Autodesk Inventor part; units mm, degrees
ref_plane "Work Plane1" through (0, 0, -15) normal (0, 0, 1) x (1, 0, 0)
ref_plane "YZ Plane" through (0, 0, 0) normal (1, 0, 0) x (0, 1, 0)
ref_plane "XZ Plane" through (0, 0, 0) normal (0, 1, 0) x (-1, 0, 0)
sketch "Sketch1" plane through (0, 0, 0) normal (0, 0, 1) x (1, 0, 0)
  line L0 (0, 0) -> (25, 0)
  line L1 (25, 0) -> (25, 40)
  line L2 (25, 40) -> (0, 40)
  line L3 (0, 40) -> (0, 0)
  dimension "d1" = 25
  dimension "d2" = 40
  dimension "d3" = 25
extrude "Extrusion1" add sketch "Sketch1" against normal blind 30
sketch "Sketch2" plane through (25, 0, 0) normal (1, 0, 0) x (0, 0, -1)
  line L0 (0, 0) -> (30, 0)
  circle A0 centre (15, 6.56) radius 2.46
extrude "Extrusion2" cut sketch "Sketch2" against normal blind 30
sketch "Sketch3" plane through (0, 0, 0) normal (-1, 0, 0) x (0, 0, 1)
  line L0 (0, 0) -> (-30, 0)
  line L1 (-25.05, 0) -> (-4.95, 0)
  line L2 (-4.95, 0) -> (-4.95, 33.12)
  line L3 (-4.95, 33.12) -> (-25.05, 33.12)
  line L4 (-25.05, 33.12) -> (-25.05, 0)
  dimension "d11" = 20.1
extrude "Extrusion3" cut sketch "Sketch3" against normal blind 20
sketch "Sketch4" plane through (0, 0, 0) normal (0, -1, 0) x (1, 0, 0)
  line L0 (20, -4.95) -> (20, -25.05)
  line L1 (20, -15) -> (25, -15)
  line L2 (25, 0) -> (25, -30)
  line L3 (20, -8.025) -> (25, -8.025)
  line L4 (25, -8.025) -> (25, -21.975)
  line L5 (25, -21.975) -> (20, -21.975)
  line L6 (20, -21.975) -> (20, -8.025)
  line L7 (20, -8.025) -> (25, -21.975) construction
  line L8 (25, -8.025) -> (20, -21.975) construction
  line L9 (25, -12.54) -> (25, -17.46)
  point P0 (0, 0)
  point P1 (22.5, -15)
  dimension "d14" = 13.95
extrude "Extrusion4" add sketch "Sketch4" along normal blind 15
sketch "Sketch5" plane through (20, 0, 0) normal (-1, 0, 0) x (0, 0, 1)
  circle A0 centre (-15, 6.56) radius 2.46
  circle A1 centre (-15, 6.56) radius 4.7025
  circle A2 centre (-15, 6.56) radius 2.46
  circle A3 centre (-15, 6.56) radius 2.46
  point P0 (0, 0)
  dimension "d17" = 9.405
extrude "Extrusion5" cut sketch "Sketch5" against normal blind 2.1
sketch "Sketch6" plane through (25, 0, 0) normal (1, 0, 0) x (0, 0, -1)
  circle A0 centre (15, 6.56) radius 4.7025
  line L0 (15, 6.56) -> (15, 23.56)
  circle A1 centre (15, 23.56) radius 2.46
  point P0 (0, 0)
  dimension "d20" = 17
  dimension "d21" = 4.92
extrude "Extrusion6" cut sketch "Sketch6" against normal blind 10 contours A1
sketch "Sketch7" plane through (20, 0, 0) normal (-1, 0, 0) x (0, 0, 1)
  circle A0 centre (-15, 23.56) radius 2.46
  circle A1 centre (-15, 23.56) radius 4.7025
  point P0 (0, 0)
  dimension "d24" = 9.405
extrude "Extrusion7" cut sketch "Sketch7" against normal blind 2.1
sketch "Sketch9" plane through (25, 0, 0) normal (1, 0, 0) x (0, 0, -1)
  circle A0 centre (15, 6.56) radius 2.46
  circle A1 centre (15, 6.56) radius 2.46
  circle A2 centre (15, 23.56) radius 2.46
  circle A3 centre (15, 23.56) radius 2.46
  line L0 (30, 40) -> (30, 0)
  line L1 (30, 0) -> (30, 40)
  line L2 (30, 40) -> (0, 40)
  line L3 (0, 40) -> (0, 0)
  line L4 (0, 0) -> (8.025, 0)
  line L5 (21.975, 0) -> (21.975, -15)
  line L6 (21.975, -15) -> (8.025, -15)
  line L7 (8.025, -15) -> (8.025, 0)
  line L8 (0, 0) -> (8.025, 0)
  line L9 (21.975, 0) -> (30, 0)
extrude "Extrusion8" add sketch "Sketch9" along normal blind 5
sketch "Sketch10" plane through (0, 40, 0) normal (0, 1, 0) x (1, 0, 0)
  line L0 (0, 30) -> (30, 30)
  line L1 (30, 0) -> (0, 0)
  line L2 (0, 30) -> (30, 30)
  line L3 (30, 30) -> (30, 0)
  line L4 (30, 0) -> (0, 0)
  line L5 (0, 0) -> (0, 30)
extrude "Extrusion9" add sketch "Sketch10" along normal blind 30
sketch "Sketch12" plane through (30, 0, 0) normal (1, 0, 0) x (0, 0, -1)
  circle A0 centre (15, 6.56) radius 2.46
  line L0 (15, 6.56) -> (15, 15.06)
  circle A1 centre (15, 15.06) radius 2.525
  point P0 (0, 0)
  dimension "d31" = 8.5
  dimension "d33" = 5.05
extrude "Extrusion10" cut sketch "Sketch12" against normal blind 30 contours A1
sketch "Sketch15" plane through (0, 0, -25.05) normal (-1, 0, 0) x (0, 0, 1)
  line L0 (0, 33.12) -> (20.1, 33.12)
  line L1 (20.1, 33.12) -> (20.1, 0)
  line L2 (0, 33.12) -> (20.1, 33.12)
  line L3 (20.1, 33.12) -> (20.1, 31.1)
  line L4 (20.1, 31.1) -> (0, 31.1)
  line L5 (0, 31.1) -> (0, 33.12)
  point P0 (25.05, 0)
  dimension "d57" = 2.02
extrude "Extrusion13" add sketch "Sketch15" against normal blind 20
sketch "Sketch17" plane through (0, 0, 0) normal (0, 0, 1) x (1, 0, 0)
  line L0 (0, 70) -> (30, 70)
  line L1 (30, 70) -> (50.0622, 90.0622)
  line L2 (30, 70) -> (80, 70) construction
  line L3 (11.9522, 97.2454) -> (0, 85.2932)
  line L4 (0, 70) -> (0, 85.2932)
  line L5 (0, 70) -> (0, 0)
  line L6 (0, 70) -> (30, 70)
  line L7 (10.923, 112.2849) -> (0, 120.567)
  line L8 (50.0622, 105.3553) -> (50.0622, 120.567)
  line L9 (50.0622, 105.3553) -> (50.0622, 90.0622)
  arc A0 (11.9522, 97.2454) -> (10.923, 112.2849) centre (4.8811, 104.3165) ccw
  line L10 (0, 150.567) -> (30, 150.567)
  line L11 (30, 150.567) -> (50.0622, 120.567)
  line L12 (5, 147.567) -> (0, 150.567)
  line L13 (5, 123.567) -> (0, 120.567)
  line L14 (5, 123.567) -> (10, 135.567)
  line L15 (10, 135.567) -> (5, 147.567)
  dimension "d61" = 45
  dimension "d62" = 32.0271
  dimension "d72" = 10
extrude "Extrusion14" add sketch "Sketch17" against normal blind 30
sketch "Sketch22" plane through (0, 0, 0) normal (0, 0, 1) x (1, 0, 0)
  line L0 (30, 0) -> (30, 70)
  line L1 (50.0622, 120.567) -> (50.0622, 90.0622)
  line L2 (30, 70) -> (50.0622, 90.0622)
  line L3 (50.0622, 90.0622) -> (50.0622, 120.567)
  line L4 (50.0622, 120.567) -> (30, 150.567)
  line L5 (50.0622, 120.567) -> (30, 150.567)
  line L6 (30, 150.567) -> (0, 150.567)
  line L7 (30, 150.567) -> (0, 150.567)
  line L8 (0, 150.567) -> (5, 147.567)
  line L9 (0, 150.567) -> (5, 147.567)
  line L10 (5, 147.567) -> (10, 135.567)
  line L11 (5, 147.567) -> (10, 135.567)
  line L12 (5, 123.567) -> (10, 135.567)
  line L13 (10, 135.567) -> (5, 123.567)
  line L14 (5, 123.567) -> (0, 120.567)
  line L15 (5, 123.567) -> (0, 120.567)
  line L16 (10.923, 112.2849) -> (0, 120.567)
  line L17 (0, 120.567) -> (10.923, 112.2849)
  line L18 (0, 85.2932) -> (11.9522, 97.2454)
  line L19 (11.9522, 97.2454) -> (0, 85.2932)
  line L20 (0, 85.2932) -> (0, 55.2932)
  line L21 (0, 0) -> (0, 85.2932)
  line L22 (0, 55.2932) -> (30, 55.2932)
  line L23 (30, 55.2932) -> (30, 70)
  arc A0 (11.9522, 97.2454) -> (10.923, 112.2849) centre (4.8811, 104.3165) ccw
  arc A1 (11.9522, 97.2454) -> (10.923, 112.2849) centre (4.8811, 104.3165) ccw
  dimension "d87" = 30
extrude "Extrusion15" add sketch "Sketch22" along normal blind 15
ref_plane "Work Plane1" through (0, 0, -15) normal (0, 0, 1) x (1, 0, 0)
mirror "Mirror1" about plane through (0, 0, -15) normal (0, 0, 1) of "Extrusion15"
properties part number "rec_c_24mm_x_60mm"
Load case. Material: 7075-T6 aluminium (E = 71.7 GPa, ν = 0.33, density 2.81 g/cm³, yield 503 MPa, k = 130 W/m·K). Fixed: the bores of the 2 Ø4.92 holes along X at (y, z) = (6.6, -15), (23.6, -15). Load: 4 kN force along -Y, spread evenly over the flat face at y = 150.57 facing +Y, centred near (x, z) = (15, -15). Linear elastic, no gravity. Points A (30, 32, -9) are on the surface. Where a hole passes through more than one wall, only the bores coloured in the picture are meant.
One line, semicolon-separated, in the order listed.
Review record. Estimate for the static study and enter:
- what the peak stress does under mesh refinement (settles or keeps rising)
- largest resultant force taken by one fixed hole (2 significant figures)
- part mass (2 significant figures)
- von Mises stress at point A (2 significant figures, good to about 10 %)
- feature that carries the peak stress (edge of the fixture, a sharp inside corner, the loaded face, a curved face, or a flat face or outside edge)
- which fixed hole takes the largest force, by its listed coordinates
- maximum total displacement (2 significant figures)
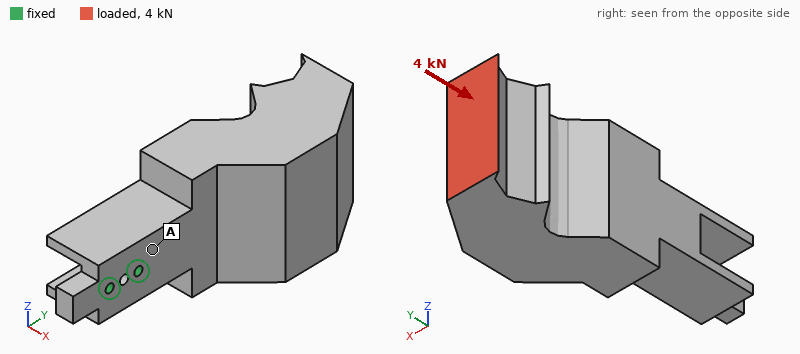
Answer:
keeps rising; 3.0 kN; 690 g; 8.8 MPa; edge of the fixture; (23.6, -15); 0.13 mm
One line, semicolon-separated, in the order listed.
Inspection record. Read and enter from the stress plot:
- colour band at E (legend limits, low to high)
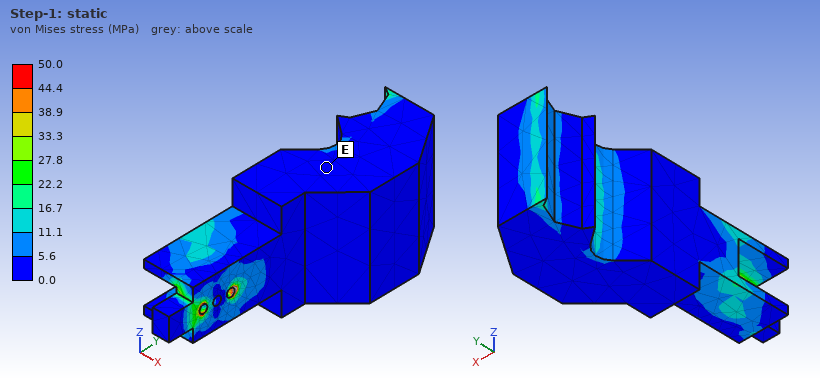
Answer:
0.0 to 5.6 MPa
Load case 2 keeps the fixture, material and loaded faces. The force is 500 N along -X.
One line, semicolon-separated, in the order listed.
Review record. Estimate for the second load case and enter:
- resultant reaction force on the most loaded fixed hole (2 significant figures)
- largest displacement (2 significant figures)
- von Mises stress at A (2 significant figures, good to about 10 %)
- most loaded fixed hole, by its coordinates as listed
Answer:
3.1 kN; 0.23 mm; 21 MPa; (23.6, -15)
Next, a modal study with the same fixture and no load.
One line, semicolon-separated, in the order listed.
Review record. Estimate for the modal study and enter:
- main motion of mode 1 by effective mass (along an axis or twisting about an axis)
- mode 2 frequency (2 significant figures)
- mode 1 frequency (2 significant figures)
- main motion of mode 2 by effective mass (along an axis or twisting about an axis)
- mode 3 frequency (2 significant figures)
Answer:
along X; 550 Hz; 480 Hz; along Z; 1300 Hz
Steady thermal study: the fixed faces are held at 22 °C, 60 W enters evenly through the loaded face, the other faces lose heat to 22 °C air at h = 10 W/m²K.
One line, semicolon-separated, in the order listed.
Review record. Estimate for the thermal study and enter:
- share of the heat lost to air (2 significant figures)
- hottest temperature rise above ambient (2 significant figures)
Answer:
15 %; 55 K
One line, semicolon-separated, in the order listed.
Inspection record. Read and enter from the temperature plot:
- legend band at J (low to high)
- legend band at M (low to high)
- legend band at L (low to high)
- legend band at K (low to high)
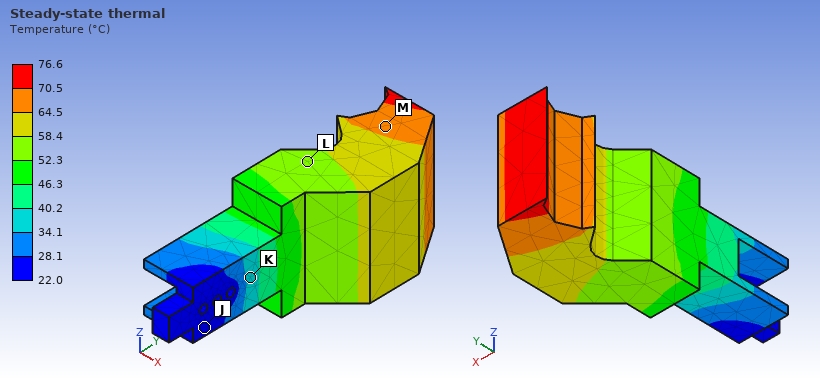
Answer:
22.0 to 28.1 °C; 64.5 to 70.5 °C; 52.3 to 58.4 °C; 34.1 to 40.2 °C
